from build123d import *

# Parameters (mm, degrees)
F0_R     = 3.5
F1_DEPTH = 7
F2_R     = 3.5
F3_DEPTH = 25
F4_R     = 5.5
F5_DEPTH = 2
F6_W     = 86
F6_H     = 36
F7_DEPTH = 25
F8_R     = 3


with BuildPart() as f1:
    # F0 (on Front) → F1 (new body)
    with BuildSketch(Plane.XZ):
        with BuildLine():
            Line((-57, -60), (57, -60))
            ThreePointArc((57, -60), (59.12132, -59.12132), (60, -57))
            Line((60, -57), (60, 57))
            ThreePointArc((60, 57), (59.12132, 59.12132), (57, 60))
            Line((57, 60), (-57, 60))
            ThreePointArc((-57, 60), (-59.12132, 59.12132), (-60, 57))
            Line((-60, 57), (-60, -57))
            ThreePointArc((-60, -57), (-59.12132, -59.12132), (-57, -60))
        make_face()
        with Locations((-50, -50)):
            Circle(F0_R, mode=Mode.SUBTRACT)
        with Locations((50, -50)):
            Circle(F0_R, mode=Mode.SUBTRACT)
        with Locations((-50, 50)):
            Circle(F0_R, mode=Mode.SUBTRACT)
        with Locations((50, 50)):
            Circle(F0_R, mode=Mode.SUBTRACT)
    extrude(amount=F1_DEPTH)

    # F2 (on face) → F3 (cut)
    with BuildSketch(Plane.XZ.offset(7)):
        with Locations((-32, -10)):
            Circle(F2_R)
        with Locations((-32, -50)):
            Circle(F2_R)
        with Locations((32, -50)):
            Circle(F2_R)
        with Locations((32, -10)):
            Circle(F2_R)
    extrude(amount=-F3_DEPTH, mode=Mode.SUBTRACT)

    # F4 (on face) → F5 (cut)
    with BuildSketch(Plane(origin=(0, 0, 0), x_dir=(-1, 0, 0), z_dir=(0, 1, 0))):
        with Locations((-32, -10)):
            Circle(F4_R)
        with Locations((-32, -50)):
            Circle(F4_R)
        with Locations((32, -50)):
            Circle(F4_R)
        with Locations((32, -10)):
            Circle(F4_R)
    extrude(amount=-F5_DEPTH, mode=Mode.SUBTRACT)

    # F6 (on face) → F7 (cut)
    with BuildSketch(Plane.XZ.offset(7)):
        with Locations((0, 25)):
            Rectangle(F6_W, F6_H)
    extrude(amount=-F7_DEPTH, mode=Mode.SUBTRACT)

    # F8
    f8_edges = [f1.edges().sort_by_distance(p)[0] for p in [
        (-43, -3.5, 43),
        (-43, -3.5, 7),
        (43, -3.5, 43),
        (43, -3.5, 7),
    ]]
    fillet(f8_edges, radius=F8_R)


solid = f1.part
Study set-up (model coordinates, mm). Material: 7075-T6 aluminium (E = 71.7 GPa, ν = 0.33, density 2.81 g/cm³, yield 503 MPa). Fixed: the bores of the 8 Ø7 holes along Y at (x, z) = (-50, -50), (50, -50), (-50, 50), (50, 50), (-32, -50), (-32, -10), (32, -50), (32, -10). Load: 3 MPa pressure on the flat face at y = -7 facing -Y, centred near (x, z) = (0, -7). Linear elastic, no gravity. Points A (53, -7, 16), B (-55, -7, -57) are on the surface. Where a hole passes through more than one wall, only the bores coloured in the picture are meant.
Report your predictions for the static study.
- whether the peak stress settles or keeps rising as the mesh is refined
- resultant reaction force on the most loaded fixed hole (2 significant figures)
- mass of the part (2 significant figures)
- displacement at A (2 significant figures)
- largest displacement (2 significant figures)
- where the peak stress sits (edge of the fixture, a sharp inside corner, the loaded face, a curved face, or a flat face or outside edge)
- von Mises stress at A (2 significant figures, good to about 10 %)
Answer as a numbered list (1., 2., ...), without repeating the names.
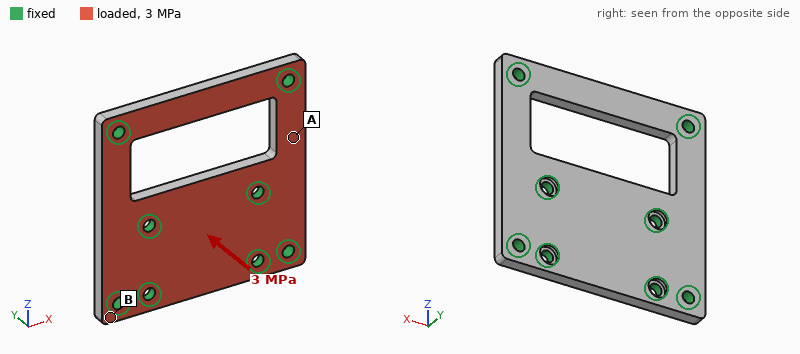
1. keeps rising
2. 6.9 kN
3. 220 g
4. 0.085 mm
5. 0.33 mm
6. edge of the fixture
7. 55 MPa
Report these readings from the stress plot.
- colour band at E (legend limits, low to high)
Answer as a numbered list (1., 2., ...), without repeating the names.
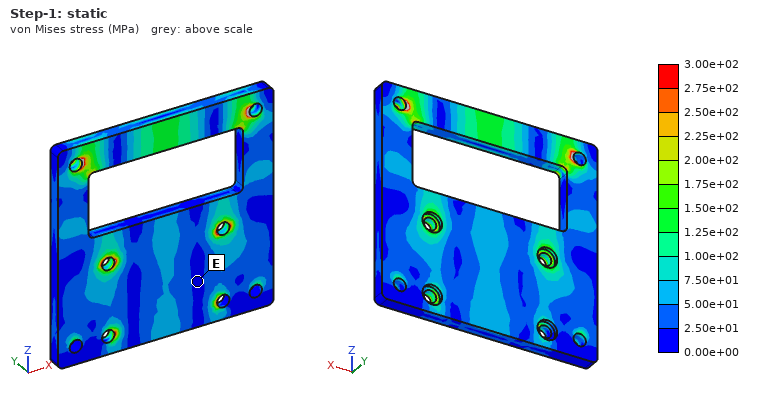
1. 0.00e+00 to 2.50e+01 MPa
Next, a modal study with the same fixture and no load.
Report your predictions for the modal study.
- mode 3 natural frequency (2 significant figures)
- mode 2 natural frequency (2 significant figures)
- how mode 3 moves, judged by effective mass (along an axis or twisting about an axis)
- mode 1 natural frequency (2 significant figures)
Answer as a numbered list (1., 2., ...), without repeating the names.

1. 6900 Hz
2. 6600 Hz
3. twisting about Z
4. 3900 Hz
